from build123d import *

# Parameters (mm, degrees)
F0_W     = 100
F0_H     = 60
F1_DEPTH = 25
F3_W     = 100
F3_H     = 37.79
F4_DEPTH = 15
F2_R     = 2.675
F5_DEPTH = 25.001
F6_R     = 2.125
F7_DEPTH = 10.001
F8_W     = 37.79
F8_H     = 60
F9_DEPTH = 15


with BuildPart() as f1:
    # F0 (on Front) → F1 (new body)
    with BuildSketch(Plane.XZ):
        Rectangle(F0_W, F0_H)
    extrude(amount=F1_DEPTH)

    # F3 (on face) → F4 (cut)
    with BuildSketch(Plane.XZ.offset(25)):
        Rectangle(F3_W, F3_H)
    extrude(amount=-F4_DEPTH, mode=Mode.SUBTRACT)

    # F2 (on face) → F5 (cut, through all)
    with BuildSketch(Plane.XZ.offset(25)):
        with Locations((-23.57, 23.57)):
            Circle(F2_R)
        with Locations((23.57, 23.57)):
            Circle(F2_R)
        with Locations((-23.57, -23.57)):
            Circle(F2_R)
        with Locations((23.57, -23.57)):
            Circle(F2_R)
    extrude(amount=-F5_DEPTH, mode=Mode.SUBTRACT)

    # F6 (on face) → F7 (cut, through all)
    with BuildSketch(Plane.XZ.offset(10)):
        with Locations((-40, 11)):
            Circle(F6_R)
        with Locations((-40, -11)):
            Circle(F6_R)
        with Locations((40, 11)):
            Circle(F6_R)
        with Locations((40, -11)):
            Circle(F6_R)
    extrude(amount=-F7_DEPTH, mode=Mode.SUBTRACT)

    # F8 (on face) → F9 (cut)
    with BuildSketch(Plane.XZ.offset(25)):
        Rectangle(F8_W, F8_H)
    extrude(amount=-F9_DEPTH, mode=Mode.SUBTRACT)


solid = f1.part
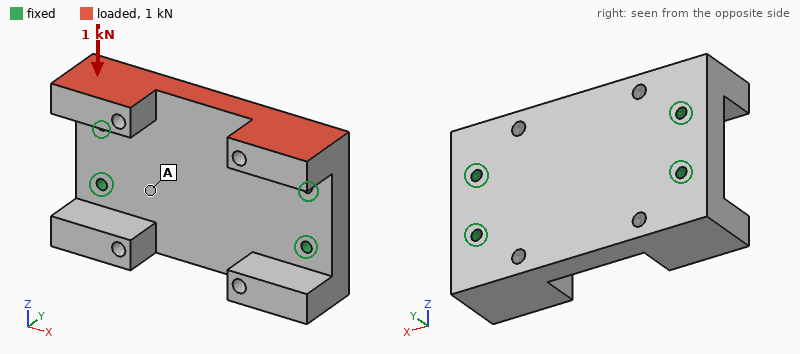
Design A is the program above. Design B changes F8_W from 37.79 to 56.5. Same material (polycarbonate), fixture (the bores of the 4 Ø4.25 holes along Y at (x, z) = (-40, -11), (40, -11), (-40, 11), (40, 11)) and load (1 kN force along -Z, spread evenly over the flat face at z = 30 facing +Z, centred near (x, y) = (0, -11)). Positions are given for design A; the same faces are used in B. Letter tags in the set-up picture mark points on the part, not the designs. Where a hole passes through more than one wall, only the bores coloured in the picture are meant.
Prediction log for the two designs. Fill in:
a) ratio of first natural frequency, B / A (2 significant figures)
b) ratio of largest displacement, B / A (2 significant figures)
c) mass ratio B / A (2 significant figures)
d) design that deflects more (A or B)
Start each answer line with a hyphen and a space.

- 1.1
- 0.90
- 0.94
- A
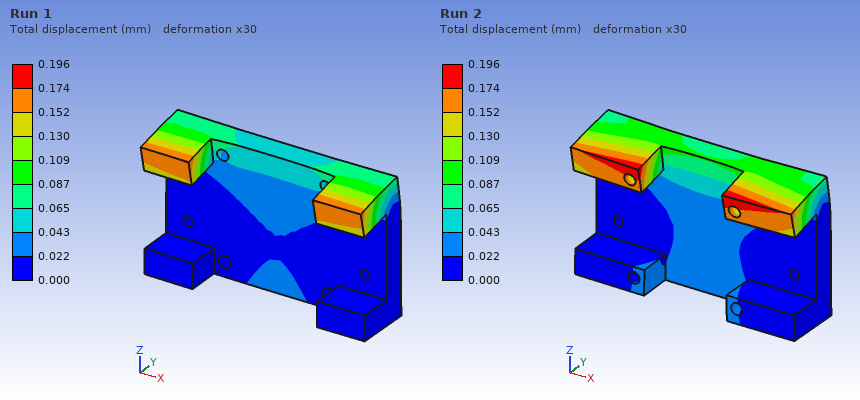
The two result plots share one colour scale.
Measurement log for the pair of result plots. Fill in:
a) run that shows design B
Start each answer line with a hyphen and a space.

- Run 1
